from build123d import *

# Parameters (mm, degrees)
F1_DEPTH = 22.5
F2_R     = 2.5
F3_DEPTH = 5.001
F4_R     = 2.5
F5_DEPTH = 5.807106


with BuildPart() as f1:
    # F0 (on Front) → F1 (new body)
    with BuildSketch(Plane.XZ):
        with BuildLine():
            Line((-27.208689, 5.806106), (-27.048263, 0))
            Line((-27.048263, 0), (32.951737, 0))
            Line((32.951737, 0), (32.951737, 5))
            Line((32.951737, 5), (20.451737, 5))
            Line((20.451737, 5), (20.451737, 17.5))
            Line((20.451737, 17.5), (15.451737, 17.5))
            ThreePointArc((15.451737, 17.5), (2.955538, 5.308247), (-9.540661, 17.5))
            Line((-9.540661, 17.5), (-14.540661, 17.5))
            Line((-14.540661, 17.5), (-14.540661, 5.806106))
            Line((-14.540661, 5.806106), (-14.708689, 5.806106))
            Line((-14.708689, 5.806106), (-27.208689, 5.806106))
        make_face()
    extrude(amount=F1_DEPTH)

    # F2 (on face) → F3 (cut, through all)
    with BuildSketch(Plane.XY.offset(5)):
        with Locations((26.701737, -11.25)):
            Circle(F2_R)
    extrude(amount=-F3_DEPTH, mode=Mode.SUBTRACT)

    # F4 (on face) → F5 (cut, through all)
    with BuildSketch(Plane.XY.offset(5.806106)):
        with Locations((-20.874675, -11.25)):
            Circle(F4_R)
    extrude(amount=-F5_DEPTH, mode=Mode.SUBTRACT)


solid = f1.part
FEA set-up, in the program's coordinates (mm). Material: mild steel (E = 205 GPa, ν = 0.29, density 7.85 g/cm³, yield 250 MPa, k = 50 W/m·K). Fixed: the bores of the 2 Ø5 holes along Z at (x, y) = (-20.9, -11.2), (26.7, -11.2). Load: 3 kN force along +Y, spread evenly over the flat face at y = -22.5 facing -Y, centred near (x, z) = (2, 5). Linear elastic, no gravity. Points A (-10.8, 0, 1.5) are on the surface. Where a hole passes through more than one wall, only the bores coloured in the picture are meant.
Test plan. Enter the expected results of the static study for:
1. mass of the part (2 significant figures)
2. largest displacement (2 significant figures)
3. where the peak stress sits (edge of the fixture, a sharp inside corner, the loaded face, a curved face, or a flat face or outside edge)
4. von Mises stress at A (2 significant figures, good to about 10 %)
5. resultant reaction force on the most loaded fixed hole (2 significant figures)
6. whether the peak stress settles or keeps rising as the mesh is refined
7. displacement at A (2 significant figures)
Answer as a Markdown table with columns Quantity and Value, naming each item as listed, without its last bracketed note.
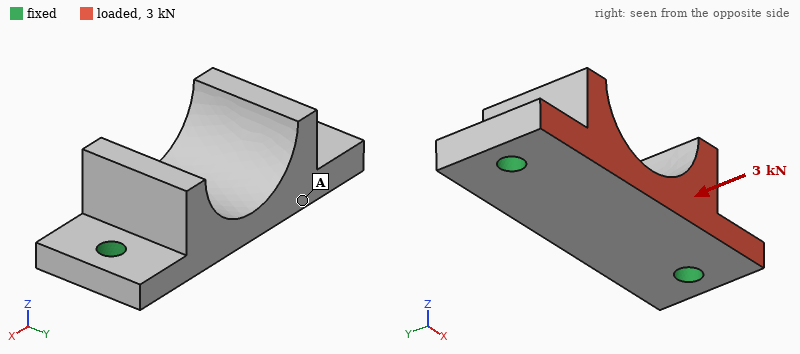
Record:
| Quantity | Value |
|---|---|
| mass of the part | 88 g |
| largest displacement | 9.1 µm |
| where the peak stress sits | edge of the fixture |
| von Mises stress at A | 15 MPa |
| resultant reaction force on the most loaded fixed hole | 1.5 kN |
| whether the peak stress settles or keeps rising as the mesh is refined | keeps rising |
| displacement at A | 3.8 µm |
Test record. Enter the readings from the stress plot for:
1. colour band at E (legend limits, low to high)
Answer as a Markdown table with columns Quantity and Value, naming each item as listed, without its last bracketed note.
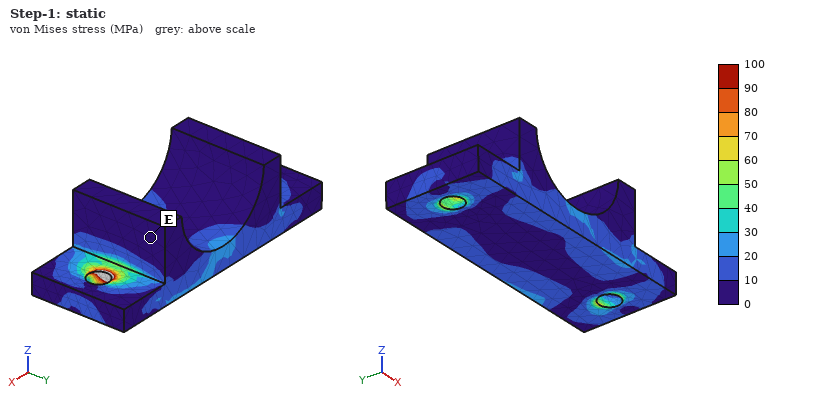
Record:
| Quantity | Value |
|---|---|
| colour band at E | 0 to 10 MPa |
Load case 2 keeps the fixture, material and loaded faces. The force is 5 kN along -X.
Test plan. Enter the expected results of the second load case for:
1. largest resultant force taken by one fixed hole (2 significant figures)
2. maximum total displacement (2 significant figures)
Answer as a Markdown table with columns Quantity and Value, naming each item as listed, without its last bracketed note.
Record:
| Quantity | Value |
|---|---|
| largest resultant force taken by one fixed hole | 2.9 kN |
| maximum total displacement | 8.0 µm |
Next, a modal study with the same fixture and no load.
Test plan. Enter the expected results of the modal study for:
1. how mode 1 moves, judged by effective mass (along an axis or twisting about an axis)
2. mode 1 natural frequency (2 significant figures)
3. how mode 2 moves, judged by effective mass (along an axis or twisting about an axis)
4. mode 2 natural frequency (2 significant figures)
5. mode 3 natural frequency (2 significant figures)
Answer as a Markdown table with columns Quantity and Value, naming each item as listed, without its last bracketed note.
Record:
| Quantity | Value |
|---|---|
| how mode 1 moves, judged by effective mass | along Z |
| mode 1 natural frequency | 9200 Hz |
| how mode 2 moves, judged by effective mass | along Y |
| mode 2 natural frequency | 10 kHz |
| mode 3 natural frequency | 17 kHz |
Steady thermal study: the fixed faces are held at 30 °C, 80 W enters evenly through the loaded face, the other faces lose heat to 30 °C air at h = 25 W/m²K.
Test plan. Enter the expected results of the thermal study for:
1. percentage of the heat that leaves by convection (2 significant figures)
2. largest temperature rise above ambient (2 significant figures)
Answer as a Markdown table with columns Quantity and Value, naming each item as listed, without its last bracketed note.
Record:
| Quantity | Value |
|---|---|
| percentage of the heat that leaves by convection | 5.9 % |
| largest temperature rise above ambient | 87 K |
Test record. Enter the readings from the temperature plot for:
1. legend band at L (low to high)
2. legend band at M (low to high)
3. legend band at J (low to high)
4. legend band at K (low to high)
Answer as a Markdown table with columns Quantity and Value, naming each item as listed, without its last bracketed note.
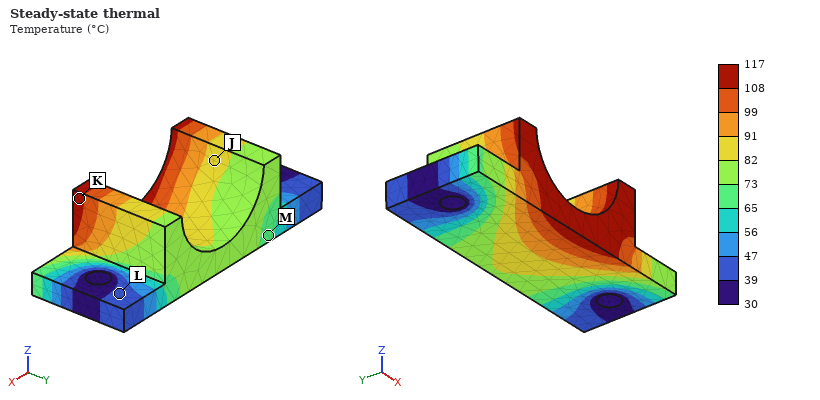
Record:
| Quantity | Value |
|---|---|
| legend band at L | 39 to 47 °C |
| legend band at M | 65 to 73 °C |
| legend band at J | 82 to 91 °C |
| legend band at K | 108 to 117 °C |
